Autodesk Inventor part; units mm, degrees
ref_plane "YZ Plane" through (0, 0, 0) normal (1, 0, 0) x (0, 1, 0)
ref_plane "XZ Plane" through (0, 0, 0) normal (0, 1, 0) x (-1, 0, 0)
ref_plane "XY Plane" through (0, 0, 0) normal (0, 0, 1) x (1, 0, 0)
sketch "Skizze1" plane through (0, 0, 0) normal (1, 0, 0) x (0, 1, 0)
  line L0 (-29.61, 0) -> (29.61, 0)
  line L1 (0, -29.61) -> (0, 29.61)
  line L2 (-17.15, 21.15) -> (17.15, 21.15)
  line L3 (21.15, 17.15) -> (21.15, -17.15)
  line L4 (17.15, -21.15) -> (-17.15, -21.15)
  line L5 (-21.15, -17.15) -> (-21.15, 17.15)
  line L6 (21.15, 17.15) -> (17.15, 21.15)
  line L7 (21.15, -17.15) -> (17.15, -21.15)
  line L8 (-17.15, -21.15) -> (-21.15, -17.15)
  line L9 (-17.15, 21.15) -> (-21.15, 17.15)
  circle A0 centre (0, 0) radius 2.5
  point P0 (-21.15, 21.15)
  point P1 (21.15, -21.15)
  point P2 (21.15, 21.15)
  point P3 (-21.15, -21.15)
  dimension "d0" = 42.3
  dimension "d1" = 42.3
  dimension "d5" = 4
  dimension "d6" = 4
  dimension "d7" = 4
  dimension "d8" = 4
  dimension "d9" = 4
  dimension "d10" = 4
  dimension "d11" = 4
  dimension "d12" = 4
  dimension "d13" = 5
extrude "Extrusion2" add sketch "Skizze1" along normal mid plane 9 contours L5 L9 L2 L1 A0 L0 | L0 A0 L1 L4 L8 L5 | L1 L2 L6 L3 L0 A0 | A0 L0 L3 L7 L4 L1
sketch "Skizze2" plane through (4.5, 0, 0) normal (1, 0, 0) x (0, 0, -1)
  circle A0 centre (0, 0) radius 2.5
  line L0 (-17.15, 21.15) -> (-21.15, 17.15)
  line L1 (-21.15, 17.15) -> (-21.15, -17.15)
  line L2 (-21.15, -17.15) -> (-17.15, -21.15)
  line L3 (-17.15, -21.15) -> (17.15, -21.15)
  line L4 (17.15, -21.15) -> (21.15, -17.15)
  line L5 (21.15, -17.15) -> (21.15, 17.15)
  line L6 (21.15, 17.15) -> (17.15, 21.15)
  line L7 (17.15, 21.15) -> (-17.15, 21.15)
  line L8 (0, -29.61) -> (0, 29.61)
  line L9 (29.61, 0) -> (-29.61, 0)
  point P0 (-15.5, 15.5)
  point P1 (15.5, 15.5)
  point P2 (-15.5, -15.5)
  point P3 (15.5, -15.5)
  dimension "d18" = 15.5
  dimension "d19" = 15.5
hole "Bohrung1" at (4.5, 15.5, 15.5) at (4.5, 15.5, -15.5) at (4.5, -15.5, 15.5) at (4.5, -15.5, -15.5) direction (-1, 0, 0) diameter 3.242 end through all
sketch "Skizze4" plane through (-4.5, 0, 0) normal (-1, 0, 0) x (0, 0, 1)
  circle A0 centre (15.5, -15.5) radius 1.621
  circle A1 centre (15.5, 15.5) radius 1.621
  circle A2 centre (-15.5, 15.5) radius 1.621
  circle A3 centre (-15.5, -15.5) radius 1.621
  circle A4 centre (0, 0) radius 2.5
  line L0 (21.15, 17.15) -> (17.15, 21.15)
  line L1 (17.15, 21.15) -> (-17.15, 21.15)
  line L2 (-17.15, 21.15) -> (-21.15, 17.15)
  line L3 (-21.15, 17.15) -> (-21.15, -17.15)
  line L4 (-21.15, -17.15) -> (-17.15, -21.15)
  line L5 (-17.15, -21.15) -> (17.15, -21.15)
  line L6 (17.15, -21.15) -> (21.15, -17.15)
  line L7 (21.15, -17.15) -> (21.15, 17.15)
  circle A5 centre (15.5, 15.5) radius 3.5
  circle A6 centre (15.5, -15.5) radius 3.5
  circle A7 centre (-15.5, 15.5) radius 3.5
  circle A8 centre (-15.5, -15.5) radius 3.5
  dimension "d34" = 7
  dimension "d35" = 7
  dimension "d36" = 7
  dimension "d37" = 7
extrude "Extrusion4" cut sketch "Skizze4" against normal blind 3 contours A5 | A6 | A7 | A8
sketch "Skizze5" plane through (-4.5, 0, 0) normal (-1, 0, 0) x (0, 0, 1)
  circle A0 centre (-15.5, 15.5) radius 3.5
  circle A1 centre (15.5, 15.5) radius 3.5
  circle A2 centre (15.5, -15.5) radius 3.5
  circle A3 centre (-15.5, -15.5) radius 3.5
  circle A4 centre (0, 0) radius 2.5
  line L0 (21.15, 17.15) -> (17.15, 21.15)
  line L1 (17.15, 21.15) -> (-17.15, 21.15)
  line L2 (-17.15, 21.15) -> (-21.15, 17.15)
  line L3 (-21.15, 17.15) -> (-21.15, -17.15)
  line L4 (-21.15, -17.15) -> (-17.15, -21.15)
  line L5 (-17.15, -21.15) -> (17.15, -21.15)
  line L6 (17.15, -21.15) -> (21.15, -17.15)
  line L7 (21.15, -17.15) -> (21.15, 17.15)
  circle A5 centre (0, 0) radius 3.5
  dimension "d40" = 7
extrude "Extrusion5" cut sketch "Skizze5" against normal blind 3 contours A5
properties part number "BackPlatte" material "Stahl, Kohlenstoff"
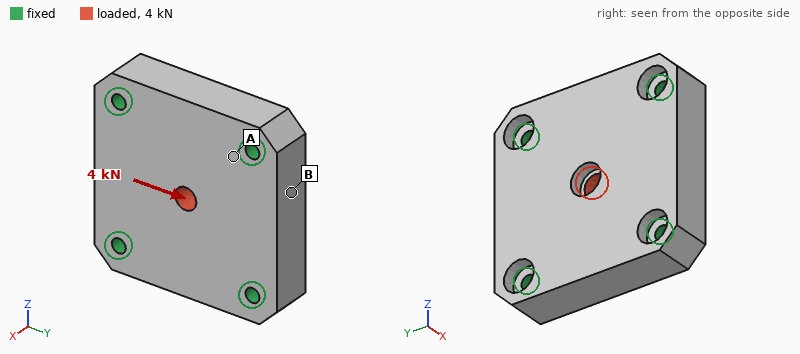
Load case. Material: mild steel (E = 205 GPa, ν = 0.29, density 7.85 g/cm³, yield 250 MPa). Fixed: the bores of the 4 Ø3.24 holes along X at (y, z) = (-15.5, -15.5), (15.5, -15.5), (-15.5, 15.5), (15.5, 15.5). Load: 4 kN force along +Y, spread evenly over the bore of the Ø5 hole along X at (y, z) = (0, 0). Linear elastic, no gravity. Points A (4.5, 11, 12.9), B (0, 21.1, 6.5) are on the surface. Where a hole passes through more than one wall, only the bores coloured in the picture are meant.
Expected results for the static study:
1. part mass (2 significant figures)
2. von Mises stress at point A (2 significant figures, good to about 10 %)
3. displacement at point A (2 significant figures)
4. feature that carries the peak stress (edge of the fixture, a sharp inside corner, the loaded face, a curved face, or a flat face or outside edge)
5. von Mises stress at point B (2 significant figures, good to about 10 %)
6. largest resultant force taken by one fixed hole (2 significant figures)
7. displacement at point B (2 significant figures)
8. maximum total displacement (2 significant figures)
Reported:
120 g
18 MPa
0.38 µm
a sharp inside corner
7.7 MPa
1.1 kN
0.93 µm
2.4 µm
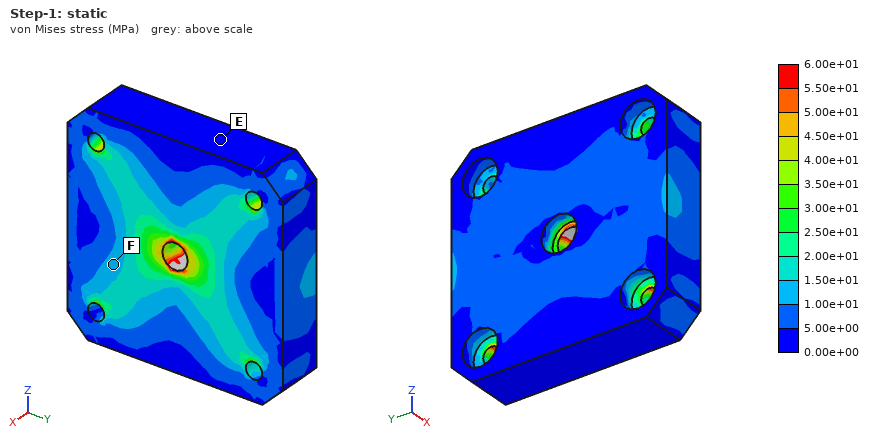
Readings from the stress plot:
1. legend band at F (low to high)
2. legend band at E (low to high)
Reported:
1.00e+01 to 1.50e+01 MPa
0.00e+00 to 5.00e+00 MPa
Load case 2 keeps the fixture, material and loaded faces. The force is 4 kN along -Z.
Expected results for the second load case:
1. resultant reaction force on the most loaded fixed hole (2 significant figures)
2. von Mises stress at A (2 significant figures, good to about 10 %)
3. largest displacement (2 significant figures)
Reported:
1.1 kN
17 MPa
2.4 µm
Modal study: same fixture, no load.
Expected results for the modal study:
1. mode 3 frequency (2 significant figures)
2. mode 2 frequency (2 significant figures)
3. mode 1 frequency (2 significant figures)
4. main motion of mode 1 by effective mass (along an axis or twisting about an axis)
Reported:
31 kHz
31 kHz
21 kHz
along X
